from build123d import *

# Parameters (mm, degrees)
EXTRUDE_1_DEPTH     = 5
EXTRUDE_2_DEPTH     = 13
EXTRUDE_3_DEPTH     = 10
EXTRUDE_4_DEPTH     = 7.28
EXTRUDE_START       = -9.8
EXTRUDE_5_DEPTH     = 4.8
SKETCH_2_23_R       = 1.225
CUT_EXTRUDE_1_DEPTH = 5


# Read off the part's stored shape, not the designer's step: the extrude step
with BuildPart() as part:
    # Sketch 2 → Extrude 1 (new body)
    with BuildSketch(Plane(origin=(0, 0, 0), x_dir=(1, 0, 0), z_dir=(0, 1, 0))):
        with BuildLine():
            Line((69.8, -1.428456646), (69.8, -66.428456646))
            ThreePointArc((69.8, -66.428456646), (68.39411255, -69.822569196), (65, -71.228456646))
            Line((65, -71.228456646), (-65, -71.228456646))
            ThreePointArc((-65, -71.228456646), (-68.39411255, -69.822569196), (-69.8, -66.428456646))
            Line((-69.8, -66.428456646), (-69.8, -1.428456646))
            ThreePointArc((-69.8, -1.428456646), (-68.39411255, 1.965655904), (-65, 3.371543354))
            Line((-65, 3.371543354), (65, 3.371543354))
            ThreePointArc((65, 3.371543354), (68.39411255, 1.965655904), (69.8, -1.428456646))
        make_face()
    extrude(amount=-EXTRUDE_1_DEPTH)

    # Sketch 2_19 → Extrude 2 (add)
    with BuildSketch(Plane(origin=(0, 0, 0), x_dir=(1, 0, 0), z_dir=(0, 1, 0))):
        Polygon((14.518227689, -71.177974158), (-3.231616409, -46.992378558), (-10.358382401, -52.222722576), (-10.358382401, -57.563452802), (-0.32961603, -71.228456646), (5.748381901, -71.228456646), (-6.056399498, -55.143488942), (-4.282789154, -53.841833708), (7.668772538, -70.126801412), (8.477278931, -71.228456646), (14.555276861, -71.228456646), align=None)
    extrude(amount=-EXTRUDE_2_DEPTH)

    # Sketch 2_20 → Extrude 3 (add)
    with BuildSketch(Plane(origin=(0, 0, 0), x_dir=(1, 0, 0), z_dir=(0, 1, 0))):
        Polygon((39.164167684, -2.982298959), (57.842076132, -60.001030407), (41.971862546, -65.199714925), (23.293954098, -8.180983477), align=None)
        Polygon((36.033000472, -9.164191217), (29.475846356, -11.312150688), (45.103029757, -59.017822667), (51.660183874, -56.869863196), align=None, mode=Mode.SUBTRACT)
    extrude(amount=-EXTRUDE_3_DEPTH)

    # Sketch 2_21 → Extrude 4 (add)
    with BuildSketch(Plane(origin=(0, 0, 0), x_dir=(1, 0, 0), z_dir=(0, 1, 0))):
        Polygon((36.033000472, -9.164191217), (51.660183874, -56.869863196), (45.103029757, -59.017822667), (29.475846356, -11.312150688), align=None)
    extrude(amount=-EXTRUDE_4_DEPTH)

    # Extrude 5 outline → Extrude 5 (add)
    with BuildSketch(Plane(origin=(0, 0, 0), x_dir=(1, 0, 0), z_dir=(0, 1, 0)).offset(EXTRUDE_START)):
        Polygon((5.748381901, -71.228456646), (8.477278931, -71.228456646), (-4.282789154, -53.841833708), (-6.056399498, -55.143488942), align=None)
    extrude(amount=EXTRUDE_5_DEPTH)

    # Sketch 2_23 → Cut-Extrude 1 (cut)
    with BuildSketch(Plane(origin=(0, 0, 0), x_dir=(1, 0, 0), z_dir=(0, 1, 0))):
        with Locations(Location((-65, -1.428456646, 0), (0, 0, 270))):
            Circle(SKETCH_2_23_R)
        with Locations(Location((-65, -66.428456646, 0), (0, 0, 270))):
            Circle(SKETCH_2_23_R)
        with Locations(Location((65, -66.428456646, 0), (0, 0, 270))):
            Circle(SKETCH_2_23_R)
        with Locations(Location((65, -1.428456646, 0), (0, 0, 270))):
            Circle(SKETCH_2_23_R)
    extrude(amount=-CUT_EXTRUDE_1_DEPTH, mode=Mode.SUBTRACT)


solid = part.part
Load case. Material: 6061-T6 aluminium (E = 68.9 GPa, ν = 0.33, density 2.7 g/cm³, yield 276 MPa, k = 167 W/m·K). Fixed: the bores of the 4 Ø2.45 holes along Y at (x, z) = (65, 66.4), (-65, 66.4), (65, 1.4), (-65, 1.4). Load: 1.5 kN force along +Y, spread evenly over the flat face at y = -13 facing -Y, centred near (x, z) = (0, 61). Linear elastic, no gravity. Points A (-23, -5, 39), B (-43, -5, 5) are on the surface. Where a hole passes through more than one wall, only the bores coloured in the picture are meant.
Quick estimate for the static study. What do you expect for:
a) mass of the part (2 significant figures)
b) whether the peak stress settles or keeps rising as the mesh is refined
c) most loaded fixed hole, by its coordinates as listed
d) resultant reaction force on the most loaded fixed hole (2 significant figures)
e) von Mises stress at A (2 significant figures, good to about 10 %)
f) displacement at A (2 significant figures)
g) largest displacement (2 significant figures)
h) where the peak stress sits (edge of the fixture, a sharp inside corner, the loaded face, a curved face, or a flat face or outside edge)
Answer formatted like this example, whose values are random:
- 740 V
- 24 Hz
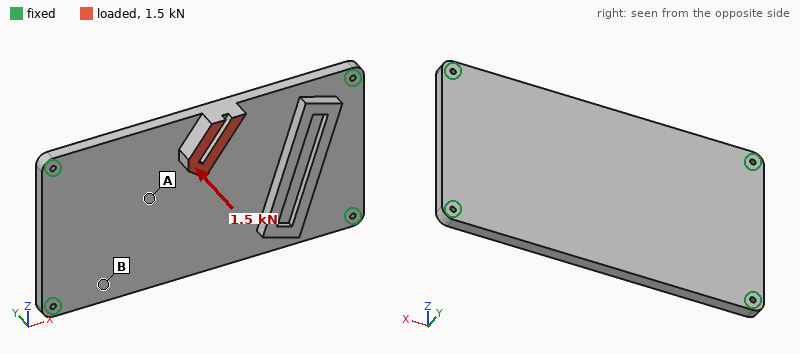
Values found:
- 160 g
- keeps rising
- (65, 66.4)
- 810 N
- 47 MPa
- 0.34 mm
- 0.65 mm
- edge of the fixture
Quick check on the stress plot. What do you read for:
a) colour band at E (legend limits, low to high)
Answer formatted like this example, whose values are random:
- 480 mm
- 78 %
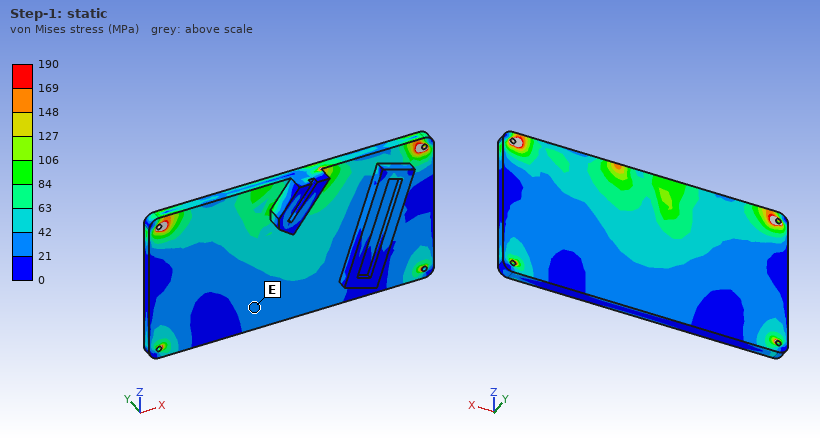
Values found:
- 21 to 42 MPa
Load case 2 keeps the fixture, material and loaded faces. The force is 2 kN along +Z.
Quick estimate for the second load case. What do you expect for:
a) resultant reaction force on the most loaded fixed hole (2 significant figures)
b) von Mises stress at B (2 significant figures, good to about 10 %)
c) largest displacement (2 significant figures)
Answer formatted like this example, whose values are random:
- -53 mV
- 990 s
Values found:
- 790 N
- 12 MPa
- 0.21 mm
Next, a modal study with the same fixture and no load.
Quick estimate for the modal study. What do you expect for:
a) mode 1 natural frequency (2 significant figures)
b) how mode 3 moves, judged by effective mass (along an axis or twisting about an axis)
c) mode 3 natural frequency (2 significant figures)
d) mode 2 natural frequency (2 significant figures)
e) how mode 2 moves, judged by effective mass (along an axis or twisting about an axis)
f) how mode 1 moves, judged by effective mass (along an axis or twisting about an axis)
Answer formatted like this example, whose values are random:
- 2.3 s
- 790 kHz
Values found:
- 1100 Hz
- twisting about Z
- 3300 Hz
- 2300 Hz
- twisting about X
- along Y
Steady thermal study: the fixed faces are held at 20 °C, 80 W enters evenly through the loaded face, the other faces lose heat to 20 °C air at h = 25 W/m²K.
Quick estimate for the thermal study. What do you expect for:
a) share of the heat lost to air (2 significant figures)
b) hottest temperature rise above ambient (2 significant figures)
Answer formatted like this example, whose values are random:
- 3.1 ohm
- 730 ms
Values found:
- 20 %
- 79 K
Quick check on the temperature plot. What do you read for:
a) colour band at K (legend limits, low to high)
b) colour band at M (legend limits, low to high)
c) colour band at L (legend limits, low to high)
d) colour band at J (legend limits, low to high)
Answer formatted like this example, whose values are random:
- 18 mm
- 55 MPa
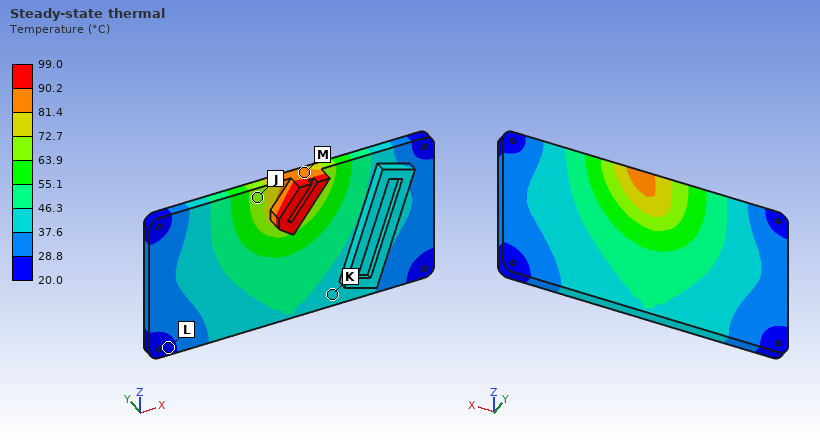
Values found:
- 37.6 to 46.3 °C
- 81.4 to 90.2 °C
- 20.0 to 28.8 °C
- 63.9 to 72.7 °C
